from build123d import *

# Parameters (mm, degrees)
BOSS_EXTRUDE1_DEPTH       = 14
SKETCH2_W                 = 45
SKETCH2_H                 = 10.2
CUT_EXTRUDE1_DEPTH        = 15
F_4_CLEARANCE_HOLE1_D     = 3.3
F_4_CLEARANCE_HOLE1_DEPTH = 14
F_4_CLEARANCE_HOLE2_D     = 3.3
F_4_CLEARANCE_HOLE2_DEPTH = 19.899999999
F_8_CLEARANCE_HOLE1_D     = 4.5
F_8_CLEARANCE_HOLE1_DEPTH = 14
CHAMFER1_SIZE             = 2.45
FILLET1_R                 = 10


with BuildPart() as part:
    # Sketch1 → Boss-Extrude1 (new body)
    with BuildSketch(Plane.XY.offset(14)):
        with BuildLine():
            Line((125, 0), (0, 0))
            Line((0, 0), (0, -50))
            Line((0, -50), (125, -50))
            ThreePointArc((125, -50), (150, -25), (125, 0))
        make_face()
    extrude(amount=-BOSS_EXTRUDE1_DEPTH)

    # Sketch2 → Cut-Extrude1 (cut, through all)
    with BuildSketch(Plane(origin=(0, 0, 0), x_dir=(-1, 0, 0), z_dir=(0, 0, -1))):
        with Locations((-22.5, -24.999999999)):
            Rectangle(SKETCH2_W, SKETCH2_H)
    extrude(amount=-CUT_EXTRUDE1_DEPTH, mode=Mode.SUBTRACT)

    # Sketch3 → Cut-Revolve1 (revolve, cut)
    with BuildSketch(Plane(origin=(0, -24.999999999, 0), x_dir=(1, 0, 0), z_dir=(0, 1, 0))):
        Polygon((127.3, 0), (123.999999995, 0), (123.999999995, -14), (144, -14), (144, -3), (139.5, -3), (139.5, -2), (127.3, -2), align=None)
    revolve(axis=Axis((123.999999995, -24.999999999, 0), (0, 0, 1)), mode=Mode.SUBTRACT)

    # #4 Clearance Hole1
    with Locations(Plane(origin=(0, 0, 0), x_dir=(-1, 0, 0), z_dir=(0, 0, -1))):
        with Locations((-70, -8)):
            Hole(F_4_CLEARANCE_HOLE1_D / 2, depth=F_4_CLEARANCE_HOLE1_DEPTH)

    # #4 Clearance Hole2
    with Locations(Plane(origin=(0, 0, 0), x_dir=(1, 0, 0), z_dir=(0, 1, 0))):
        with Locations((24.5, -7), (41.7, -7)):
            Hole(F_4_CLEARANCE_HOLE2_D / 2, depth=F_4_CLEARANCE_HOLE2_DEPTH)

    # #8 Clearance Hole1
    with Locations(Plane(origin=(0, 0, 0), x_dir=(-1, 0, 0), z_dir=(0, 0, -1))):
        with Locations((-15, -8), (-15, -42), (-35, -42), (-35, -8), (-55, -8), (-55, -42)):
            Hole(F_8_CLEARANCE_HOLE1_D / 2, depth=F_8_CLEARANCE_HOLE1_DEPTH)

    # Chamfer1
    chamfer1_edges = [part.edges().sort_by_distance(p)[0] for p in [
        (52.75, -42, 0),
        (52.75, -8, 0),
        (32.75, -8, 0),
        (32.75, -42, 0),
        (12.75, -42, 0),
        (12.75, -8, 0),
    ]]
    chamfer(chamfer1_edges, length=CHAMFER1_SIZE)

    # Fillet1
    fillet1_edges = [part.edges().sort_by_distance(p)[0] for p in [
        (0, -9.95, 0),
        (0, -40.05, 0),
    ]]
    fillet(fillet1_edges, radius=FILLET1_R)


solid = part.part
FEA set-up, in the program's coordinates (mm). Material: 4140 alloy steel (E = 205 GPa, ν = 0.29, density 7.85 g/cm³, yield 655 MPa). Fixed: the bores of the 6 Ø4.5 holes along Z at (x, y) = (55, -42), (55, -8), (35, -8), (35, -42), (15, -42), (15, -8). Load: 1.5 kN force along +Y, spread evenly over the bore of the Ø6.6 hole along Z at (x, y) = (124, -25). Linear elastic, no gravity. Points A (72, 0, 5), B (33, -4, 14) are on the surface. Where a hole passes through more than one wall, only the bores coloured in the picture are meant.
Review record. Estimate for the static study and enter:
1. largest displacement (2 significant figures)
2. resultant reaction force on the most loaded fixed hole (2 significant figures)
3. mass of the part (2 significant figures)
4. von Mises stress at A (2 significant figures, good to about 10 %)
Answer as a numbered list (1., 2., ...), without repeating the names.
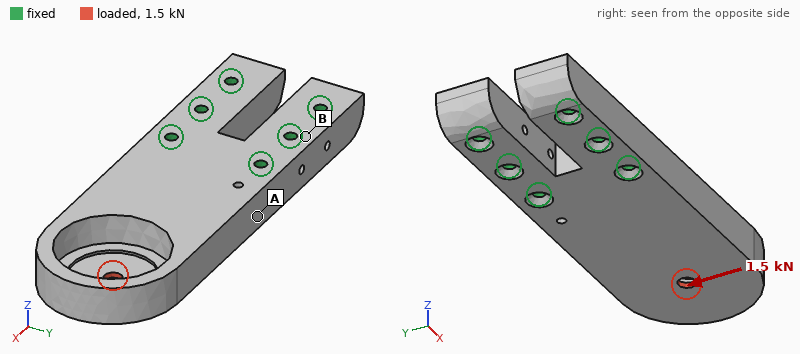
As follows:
1. 15 µm
2. 2.6 kN
3. 610 g
4. 13 MPa
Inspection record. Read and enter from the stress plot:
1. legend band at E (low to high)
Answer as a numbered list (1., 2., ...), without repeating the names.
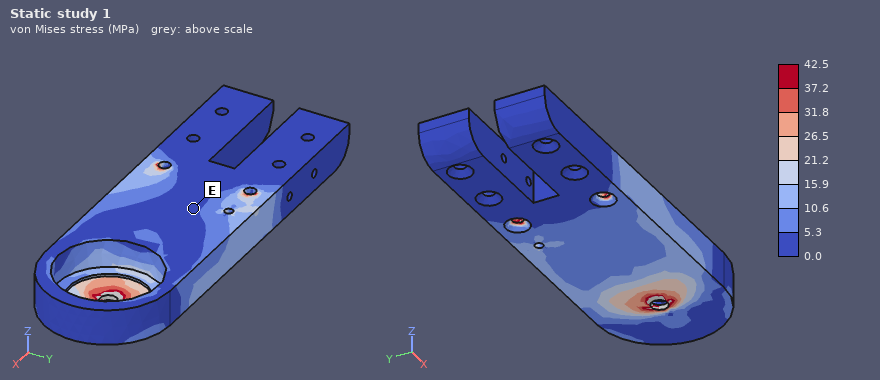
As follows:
1. 0.0 to 5.3 MPa
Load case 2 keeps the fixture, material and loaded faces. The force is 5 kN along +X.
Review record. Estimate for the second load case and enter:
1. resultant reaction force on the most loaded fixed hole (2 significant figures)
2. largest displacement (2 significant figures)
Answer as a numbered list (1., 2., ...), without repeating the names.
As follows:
1. 2.0 kN
2. 62 µm
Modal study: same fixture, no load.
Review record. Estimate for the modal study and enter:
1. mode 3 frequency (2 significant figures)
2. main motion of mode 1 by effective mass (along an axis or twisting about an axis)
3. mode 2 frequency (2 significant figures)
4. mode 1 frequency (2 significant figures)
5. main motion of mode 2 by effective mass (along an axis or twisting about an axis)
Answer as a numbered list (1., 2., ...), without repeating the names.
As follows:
1. 5200 Hz
2. along Z
3. 4400 Hz
4. 1700 Hz
5. along Y
